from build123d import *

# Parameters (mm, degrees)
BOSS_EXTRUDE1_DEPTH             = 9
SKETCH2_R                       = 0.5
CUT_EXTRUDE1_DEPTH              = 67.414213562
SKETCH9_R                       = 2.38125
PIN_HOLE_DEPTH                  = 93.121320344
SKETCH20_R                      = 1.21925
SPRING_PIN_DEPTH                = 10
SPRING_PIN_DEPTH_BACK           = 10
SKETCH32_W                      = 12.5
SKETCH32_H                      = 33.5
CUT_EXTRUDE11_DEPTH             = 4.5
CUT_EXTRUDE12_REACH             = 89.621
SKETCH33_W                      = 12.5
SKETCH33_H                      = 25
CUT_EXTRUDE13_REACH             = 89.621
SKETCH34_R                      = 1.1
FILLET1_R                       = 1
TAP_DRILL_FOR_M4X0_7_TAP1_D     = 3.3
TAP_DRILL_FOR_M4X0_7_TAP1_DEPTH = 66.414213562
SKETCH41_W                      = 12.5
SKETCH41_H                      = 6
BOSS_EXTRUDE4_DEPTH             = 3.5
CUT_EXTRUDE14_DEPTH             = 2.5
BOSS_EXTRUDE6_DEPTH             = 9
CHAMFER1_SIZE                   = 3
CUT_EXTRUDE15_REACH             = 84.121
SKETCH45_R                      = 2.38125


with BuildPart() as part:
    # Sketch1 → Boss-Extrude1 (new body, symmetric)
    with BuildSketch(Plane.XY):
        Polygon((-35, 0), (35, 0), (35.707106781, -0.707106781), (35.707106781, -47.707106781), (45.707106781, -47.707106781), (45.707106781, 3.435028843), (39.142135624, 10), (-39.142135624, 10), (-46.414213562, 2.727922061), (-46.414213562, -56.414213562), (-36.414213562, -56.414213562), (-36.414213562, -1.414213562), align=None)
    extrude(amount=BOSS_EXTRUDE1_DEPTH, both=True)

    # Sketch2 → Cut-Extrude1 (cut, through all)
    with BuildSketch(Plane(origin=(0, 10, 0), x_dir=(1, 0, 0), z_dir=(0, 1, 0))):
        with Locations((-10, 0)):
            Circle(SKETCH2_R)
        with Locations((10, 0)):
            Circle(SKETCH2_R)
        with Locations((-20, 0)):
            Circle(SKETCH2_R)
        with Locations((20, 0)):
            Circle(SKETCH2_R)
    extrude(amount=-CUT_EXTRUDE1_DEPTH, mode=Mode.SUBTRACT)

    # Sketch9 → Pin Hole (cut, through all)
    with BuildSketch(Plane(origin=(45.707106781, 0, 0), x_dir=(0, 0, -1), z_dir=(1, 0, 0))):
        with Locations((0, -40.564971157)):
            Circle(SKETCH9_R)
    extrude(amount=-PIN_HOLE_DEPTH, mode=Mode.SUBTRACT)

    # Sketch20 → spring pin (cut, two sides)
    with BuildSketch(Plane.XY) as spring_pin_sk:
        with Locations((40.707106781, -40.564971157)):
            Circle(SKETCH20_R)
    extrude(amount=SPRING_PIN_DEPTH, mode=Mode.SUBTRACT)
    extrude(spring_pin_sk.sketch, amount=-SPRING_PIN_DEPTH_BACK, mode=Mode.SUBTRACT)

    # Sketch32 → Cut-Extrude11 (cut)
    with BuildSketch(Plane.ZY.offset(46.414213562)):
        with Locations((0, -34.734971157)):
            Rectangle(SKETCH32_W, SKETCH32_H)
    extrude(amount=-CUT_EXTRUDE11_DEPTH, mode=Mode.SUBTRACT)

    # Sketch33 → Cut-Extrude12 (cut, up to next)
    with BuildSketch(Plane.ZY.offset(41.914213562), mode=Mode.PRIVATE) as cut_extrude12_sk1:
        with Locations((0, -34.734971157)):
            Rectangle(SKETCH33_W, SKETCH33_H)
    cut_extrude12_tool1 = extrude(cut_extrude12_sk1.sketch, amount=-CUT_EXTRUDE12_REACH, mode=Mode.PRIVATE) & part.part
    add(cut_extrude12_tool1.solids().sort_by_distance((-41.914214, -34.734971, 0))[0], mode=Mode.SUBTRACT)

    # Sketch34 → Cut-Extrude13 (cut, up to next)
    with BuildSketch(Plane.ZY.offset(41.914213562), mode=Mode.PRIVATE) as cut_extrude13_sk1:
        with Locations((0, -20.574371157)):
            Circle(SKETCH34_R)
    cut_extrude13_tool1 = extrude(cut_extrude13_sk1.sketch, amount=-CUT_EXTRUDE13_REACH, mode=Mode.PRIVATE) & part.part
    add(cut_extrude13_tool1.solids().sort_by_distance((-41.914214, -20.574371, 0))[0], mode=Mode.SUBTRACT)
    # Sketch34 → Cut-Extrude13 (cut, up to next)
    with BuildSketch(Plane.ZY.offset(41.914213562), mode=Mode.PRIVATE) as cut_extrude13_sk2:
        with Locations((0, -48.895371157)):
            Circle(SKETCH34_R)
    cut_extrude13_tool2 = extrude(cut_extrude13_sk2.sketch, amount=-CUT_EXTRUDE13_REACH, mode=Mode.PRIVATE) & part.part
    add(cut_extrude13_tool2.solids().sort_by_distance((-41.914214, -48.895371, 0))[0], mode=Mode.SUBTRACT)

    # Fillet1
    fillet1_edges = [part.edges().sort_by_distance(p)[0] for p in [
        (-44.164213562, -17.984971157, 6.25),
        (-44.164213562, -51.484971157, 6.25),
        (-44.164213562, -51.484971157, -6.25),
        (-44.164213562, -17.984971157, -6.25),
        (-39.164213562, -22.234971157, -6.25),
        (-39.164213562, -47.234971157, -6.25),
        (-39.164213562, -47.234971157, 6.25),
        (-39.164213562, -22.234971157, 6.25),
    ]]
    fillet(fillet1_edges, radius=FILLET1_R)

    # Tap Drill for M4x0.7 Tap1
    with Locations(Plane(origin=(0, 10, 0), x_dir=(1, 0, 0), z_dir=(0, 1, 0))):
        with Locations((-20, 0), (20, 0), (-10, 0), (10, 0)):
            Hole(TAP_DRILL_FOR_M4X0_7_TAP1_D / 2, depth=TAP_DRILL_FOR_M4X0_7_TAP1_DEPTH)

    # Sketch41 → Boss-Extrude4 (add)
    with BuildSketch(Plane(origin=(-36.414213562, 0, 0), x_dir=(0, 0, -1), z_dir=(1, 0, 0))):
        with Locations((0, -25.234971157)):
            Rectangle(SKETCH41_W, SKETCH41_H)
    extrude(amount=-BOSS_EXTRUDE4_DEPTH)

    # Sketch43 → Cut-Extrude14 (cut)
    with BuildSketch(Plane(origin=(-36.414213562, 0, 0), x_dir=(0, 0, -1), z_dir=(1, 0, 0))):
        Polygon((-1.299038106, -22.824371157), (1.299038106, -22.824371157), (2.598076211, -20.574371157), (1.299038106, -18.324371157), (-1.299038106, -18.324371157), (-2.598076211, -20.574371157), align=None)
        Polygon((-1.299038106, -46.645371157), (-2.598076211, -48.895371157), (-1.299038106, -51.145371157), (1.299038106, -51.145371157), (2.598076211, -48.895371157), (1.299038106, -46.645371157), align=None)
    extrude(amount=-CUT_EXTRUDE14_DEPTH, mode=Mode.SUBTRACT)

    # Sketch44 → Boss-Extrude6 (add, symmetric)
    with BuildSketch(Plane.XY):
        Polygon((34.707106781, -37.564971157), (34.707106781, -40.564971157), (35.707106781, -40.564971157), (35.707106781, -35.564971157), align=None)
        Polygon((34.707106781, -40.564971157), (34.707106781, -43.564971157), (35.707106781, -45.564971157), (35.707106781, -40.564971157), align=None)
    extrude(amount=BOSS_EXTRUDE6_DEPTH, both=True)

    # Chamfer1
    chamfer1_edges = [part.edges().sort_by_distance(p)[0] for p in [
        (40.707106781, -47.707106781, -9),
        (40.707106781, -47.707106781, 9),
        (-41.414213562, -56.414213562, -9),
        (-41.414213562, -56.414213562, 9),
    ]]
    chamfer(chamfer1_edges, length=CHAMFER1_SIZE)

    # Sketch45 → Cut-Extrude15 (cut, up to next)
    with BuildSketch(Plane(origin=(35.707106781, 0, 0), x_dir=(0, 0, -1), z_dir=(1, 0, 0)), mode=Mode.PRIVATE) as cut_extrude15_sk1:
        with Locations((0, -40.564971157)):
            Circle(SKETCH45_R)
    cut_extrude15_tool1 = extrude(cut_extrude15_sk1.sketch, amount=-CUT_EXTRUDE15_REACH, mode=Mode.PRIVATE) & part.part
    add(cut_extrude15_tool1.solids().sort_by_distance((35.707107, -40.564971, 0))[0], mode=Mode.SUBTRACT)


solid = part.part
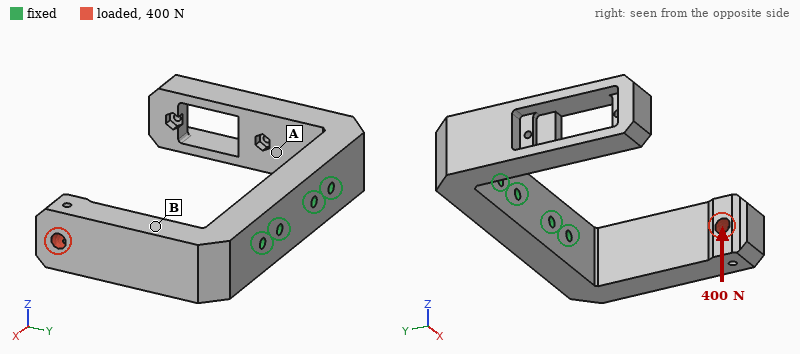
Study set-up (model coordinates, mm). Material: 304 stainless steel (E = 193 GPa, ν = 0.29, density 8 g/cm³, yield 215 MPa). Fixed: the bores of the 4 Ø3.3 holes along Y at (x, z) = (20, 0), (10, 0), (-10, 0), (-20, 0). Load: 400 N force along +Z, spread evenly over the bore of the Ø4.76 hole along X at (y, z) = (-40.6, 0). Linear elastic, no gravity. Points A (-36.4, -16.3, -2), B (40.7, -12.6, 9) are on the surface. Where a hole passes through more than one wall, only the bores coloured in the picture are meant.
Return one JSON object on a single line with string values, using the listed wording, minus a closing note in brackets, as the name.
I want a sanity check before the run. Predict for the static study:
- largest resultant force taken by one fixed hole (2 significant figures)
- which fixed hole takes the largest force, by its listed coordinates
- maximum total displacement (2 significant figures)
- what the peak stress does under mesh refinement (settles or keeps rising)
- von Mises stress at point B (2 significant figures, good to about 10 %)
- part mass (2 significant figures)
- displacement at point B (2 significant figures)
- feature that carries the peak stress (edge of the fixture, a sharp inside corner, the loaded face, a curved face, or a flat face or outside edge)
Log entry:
{"largest resultant force taken by one fixed hole": "810 N", "which fixed hole takes the largest force, by its listed coordinates": "(20, 0)", "maximum total displacement": "81 µm", "what the peak stress does under mesh refinement": "keeps rising", "von Mises stress at point B": "21 MPa", "part mass": "240 g", "displacement at point B": "28 µm", "feature that carries the peak stress": "edge of the fixture"}
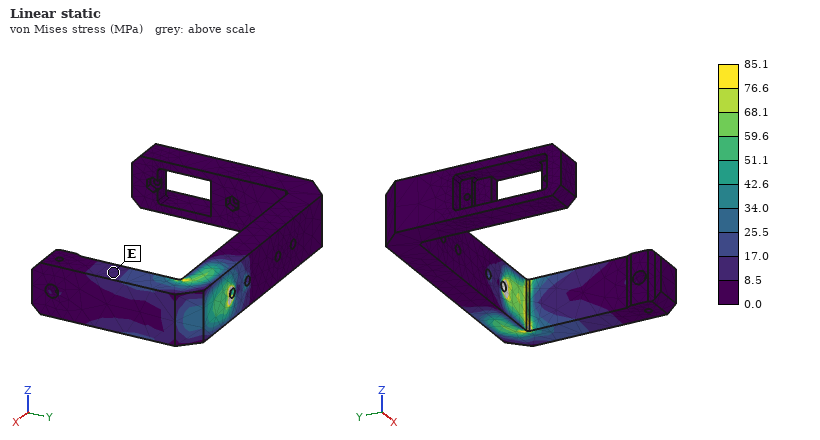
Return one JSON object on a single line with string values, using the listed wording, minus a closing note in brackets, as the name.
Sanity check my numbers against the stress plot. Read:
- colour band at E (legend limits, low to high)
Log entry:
{"colour band at E": "8.5 to 17.0 MPa"}
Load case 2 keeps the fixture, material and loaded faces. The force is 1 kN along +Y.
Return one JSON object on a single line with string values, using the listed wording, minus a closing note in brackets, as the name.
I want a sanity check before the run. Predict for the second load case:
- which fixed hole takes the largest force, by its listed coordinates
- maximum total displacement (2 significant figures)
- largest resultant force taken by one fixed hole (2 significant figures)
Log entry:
{"which fixed hole takes the largest force, by its listed coordinates": "(20, 0)", "maximum total displacement": "45 µm", "largest resultant force taken by one fixed hole": "1.4 kN"}
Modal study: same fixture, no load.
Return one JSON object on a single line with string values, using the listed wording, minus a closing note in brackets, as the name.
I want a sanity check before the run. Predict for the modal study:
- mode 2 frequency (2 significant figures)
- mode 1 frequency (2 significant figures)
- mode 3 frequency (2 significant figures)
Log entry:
{"mode 2 frequency": "1800 Hz", "mode 1 frequency": "1700 Hz", "mode 3 frequency": "1800 Hz"}
